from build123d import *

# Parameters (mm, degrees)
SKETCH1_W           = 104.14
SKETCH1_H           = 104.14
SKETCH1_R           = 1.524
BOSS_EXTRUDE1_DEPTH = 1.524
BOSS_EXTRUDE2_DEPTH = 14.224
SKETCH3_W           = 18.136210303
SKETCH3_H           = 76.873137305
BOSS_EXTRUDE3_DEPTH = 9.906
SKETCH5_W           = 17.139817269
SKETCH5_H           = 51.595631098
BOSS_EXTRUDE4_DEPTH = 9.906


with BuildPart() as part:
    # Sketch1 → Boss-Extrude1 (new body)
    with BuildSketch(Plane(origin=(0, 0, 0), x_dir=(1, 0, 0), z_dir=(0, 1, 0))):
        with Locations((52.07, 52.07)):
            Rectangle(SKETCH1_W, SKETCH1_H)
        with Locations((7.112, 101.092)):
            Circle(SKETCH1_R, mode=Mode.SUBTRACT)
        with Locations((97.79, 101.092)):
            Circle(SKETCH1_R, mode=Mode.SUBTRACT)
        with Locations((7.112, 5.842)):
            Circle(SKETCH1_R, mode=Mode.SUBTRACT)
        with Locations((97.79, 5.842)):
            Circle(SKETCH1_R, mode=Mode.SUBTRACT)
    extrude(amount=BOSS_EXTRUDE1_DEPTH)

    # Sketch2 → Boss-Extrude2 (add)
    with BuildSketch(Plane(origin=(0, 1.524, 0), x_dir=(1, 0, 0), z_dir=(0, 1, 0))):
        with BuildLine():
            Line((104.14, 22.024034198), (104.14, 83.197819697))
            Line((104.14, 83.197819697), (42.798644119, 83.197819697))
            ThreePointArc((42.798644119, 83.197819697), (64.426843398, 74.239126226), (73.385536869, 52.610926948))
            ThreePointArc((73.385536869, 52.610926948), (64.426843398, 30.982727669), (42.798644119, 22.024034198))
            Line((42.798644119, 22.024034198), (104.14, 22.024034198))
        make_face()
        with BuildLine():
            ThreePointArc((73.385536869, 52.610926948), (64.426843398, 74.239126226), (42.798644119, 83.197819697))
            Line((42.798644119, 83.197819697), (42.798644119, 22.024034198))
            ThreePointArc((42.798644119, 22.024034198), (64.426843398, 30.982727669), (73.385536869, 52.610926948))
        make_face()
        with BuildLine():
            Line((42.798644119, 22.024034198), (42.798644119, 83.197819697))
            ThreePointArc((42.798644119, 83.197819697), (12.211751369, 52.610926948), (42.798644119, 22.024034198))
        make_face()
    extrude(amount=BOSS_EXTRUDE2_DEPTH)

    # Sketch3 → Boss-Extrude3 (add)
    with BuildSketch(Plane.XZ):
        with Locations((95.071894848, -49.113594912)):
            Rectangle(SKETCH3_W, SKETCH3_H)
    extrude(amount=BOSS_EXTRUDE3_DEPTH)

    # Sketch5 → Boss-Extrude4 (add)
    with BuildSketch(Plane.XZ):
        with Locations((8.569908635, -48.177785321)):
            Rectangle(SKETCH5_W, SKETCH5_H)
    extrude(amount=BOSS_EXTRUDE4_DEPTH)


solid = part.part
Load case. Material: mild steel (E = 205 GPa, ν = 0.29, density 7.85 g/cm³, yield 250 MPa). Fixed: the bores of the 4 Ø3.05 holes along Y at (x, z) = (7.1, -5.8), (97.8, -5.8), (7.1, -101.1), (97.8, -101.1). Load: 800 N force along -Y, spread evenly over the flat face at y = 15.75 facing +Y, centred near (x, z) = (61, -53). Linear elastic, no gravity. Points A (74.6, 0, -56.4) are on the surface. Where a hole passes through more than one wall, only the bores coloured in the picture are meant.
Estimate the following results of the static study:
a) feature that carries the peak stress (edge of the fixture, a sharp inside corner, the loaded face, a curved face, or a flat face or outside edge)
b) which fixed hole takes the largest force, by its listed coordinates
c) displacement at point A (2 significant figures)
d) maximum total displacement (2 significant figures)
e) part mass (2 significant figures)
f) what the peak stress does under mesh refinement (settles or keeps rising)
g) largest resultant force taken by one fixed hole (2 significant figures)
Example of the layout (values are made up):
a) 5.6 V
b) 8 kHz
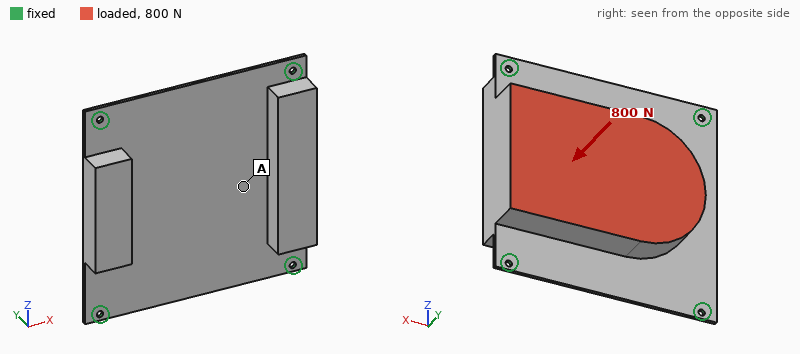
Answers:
a) edge of the fixture
b) (97.8, -101.1)
c) 0.049 mm
d) 0.11 mm
e) 890 g
f) keeps rising
g) 290 N
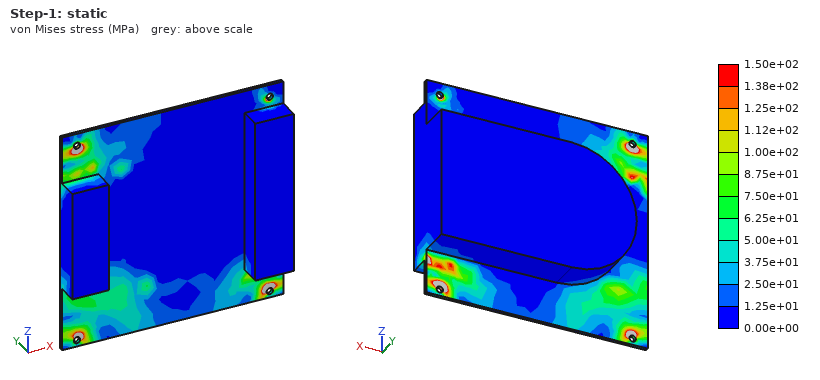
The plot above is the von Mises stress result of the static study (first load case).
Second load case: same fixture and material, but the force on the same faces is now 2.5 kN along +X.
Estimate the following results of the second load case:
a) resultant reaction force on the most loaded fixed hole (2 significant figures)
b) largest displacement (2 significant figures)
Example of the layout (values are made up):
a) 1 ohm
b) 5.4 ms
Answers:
a) 790 N
b) 0.11 mm
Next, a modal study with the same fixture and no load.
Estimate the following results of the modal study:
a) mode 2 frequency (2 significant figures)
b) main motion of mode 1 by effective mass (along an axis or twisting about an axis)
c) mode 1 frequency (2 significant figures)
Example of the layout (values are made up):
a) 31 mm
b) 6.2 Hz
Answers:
a) 1100 Hz
b) along Y
c) 590 Hz
